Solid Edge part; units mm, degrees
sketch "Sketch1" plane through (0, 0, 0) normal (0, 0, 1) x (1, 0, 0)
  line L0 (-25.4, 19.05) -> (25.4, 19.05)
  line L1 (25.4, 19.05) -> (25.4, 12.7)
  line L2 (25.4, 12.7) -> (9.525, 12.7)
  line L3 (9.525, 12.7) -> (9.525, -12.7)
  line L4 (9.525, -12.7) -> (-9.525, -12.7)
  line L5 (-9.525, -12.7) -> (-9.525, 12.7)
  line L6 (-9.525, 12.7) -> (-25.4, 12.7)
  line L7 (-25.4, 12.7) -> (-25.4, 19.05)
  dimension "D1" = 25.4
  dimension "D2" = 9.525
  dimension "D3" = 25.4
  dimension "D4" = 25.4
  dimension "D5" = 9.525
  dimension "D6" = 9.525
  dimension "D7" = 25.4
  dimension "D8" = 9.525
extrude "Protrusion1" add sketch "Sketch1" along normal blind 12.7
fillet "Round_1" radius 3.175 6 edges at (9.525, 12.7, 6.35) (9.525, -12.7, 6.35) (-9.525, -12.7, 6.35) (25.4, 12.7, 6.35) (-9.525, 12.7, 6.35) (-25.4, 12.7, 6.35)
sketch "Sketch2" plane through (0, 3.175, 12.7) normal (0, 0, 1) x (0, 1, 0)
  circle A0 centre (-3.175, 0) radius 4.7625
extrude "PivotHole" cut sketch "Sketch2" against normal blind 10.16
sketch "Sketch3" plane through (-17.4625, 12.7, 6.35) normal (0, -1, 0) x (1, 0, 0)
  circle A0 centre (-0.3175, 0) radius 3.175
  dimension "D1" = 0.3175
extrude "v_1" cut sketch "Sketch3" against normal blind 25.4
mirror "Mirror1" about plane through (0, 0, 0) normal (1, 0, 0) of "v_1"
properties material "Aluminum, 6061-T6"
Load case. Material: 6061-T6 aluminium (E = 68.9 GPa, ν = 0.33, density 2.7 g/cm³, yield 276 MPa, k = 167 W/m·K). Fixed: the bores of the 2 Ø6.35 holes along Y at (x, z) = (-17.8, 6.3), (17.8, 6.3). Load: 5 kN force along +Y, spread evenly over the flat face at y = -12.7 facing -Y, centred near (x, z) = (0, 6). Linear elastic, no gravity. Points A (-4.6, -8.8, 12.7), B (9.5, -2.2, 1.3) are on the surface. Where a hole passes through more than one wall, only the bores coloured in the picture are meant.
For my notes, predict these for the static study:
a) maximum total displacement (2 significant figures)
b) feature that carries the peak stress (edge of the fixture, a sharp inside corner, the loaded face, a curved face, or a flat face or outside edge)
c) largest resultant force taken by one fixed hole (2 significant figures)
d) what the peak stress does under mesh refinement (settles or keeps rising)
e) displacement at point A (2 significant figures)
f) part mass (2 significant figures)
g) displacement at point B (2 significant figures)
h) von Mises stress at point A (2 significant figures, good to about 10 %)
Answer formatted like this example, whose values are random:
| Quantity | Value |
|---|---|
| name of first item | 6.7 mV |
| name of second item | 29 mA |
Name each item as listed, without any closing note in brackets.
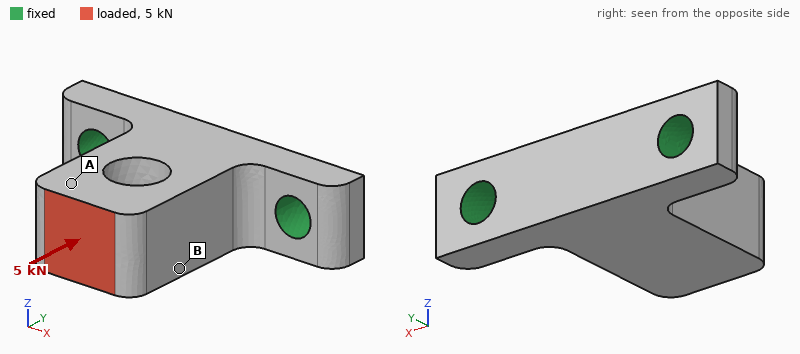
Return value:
| Quantity | Value |
|---|---|
| maximum total displacement | 34 µm |
| feature that carries the peak stress | edge of the fixture |
| largest resultant force taken by one fixed hole | 2.7 kN |
| what the peak stress does under mesh refinement | keeps rising |
| displacement at point A | 30 µm |
| part mass | 24 g |
| displacement at point B | 21 µm |
| von Mises stress at point A | 44 MPa |
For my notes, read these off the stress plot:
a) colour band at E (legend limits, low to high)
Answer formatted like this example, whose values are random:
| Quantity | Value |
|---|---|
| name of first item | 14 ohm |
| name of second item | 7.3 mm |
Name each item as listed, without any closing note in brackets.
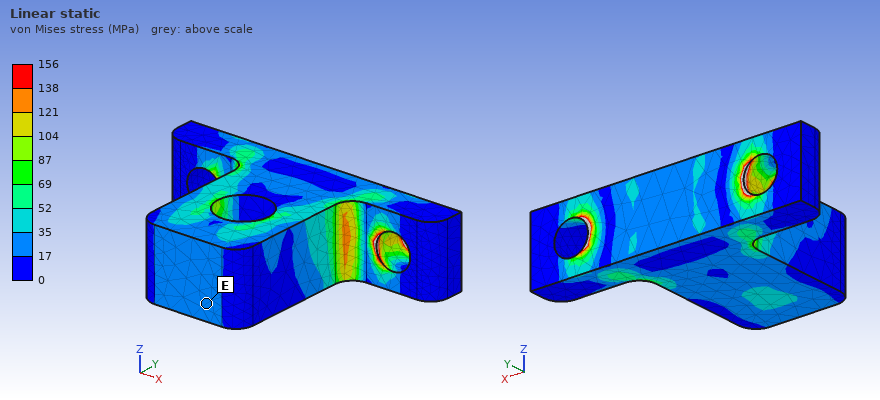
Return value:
| Quantity | Value |
|---|---|
| colour band at E | 17 to 35 MPa |
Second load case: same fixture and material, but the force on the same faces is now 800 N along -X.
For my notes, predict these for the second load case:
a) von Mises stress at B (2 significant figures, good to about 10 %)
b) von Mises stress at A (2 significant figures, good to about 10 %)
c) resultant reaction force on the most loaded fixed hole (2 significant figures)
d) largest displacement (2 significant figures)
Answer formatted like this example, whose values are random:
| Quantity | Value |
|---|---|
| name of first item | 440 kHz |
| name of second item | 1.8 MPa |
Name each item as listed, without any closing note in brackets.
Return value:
| Quantity | Value |
|---|---|
| von Mises stress at B | 8.2 MPa |
| von Mises stress at A | 9.3 MPa |
| resultant reaction force on the most loaded fixed hole | 950 N |
| largest displacement | 28 µm |
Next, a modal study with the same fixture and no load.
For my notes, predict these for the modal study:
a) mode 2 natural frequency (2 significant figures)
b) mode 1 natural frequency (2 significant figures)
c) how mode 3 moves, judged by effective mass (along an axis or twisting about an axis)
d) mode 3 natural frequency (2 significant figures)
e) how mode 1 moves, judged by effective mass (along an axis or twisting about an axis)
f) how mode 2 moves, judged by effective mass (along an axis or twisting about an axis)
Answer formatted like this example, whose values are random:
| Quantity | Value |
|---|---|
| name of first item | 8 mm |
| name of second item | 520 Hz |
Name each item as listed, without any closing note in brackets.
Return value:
| Quantity | Value |
|---|---|
| mode 2 natural frequency | 12 kHz |
| mode 1 natural frequency | 5300 Hz |
| how mode 3 moves, judged by effective mass | along Y |
| mode 3 natural frequency | 19 kHz |
| how mode 1 moves, judged by effective mass | along Z |
| how mode 2 moves, judged by effective mass | along X |
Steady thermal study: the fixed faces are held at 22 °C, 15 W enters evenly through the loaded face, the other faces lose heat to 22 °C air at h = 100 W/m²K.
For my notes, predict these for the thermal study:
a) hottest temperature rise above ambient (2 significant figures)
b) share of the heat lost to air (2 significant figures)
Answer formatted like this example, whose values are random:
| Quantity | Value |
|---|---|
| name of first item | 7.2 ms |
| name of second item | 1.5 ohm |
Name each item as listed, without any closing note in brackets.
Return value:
| Quantity | Value |
|---|---|
| hottest temperature rise above ambient | 16 K |
| share of the heat lost to air | 14 % |
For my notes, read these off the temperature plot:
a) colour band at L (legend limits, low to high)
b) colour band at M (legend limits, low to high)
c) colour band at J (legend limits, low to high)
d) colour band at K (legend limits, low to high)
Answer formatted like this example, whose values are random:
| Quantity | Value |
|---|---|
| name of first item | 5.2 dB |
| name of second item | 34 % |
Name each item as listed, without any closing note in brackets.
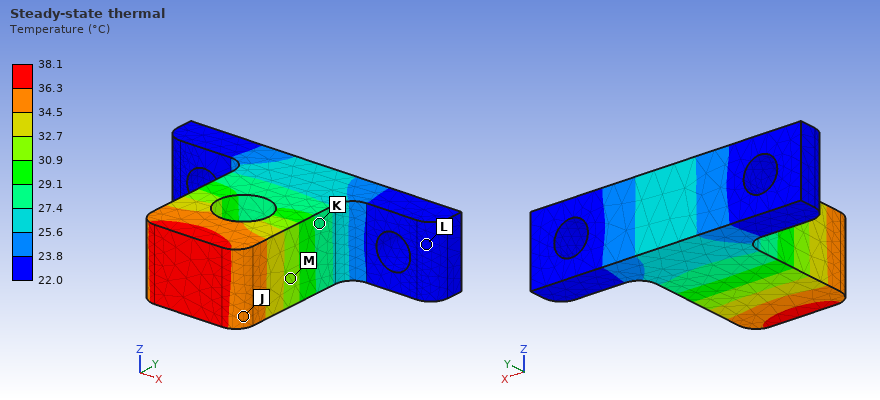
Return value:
| Quantity | Value |
|---|---|
| colour band at L | 22.0 to 23.8 °C |
| colour band at M | 30.9 to 32.7 °C |
| colour band at J | 34.5 to 36.3 °C |
| colour band at K | 27.4 to 29.1 °C |
